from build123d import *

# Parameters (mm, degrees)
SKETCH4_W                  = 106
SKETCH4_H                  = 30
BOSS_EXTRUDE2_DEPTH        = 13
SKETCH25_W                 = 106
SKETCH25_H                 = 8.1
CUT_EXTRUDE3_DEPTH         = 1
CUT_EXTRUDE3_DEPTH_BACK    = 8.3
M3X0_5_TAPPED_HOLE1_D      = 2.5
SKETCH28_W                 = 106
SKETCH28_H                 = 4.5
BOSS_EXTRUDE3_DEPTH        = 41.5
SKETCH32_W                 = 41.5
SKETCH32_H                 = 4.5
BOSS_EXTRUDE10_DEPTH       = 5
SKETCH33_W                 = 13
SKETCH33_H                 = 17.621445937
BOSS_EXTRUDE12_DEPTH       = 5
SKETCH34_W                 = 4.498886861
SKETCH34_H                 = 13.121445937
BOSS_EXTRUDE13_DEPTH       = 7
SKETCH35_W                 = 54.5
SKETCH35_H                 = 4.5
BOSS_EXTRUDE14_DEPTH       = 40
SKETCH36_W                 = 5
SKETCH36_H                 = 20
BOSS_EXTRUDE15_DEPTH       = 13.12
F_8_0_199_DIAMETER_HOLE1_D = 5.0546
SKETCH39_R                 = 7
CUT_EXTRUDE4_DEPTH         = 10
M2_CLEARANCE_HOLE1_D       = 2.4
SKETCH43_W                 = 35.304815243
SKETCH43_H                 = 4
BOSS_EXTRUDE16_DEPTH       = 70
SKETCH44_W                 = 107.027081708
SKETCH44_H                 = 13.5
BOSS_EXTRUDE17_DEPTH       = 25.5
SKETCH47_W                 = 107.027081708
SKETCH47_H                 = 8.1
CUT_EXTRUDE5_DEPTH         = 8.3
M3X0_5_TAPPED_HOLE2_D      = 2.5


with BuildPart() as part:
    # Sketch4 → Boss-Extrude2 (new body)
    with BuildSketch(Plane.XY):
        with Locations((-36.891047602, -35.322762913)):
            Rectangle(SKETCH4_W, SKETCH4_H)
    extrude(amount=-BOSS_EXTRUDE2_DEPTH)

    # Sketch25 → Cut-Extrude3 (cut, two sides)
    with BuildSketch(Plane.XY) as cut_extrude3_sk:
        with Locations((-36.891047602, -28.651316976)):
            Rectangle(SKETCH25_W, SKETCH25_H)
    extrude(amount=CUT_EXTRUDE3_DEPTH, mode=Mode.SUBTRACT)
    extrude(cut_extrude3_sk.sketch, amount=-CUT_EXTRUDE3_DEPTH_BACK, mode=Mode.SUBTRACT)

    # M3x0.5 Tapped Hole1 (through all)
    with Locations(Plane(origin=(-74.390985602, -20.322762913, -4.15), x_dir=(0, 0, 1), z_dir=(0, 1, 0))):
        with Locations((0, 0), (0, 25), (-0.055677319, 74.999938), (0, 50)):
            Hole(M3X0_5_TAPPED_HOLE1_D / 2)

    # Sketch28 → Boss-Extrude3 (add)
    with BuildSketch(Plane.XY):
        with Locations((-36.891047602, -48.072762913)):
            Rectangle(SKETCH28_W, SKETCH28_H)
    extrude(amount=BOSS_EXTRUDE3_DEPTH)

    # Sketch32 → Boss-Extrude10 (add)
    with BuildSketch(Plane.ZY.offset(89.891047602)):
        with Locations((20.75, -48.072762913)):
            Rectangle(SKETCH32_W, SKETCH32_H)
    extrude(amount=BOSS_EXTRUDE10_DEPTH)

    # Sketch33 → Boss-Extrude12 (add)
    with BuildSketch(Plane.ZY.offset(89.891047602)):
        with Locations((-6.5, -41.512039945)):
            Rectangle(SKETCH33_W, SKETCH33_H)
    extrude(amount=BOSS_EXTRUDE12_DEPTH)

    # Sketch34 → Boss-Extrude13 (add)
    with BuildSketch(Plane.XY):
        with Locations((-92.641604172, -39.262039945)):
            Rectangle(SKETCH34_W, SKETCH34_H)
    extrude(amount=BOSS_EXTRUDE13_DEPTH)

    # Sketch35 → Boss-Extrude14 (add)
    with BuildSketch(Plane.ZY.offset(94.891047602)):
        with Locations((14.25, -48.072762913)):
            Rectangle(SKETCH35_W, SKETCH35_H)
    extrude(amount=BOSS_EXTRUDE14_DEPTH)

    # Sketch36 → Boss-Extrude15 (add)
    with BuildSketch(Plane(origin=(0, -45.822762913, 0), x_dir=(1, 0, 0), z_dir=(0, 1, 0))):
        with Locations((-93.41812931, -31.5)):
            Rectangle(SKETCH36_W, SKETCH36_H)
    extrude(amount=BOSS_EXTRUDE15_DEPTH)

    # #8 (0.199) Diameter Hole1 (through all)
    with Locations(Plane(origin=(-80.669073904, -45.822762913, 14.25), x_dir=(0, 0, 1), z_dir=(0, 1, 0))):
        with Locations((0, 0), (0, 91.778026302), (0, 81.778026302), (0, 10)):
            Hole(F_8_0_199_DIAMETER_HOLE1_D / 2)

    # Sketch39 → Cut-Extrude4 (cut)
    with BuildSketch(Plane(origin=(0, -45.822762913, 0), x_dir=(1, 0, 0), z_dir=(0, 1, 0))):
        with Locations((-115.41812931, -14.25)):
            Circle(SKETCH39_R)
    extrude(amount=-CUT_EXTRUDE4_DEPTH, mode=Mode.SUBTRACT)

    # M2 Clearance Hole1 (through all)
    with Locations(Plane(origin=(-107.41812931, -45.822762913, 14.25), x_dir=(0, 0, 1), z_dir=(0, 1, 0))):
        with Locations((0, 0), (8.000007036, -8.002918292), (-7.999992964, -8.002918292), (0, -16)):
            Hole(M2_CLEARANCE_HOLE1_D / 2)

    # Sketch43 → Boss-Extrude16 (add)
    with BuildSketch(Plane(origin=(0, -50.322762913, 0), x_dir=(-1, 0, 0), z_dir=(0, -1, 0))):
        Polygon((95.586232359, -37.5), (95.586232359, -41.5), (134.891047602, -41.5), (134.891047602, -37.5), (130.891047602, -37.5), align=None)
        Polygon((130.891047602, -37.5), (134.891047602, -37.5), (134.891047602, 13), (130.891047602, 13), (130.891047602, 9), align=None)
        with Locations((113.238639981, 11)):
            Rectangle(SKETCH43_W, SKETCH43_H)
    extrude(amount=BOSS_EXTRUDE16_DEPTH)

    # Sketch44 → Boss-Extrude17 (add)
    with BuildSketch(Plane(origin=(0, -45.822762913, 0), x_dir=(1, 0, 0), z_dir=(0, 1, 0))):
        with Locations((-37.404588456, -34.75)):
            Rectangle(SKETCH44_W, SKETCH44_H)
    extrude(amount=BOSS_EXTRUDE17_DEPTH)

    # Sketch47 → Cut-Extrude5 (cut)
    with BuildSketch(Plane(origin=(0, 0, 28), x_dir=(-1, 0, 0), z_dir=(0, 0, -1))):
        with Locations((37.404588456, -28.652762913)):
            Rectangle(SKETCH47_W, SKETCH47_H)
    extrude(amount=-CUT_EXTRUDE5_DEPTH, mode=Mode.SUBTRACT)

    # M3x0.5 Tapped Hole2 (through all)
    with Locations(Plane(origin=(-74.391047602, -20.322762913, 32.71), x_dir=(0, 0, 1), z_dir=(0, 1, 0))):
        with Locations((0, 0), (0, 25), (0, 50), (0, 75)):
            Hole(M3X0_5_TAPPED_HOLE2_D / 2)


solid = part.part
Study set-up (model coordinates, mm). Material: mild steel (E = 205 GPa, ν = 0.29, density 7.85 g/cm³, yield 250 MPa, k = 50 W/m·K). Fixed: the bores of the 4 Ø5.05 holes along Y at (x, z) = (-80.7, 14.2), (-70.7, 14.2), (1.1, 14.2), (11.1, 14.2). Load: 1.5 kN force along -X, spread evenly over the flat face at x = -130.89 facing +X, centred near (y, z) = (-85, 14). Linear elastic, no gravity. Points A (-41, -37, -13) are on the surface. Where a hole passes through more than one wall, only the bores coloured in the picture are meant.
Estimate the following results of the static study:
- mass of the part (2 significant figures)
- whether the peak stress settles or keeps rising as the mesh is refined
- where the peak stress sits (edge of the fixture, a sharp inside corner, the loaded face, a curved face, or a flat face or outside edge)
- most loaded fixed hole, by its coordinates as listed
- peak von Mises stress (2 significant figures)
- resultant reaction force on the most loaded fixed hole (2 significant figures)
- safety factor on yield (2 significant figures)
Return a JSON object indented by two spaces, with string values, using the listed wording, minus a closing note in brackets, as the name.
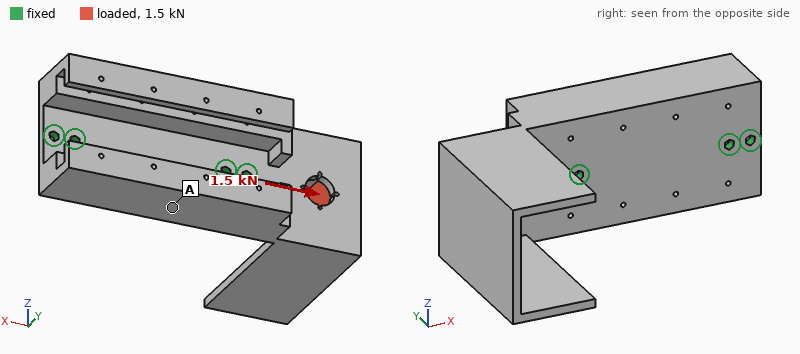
{
  "mass of the part": "1.0 kg",
  "whether the peak stress settles or keeps rising as the mesh is refined": "settles",
  "where the peak stress sits": "a flat face or outside edge",
  "most loaded fixed hole, by its coordinates as listed": "(-80.7, 14.2)",
  "peak von Mises stress": "520 MPa",
  "resultant reaction force on the most loaded fixed hole": "1.6 kN",
  "safety factor on yield": "0.48"
}
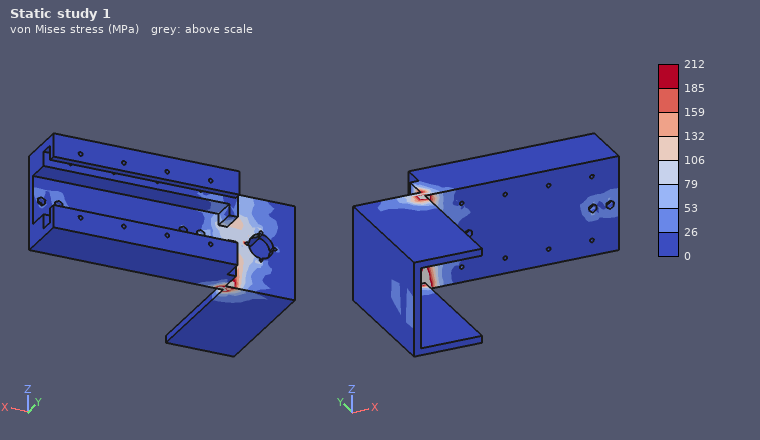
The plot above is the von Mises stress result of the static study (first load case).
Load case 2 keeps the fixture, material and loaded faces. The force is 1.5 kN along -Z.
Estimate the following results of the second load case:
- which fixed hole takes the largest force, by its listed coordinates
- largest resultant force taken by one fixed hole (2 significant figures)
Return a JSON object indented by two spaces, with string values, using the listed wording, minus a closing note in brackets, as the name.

{
  "which fixed hole takes the largest force, by its listed coordinates": "(-80.7, 14.2)",
  "largest resultant force taken by one fixed hole": "2.0 kN"
}
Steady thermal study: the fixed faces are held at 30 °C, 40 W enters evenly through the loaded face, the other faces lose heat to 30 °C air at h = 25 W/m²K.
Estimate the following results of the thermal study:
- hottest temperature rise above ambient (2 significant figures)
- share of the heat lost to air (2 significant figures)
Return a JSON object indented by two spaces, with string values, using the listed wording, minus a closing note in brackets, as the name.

{
  "hottest temperature rise above ambient": "81 K",
  "share of the heat lost to air": "73 %"
}
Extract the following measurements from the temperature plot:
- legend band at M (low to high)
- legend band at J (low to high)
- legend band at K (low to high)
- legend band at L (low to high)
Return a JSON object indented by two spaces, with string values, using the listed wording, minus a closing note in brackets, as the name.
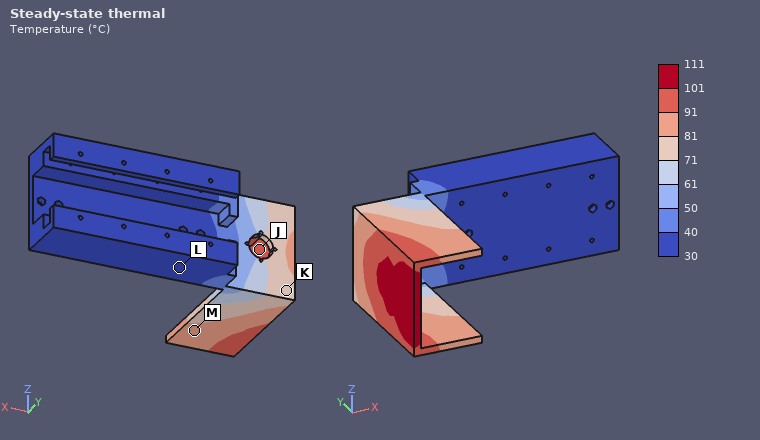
{
  "legend band at M": "81 to 91 °C",
  "legend band at J": "91 to 101 °C",
  "legend band at K": "71 to 81 °C",
  "legend band at L": "30 to 40 °C"
}
